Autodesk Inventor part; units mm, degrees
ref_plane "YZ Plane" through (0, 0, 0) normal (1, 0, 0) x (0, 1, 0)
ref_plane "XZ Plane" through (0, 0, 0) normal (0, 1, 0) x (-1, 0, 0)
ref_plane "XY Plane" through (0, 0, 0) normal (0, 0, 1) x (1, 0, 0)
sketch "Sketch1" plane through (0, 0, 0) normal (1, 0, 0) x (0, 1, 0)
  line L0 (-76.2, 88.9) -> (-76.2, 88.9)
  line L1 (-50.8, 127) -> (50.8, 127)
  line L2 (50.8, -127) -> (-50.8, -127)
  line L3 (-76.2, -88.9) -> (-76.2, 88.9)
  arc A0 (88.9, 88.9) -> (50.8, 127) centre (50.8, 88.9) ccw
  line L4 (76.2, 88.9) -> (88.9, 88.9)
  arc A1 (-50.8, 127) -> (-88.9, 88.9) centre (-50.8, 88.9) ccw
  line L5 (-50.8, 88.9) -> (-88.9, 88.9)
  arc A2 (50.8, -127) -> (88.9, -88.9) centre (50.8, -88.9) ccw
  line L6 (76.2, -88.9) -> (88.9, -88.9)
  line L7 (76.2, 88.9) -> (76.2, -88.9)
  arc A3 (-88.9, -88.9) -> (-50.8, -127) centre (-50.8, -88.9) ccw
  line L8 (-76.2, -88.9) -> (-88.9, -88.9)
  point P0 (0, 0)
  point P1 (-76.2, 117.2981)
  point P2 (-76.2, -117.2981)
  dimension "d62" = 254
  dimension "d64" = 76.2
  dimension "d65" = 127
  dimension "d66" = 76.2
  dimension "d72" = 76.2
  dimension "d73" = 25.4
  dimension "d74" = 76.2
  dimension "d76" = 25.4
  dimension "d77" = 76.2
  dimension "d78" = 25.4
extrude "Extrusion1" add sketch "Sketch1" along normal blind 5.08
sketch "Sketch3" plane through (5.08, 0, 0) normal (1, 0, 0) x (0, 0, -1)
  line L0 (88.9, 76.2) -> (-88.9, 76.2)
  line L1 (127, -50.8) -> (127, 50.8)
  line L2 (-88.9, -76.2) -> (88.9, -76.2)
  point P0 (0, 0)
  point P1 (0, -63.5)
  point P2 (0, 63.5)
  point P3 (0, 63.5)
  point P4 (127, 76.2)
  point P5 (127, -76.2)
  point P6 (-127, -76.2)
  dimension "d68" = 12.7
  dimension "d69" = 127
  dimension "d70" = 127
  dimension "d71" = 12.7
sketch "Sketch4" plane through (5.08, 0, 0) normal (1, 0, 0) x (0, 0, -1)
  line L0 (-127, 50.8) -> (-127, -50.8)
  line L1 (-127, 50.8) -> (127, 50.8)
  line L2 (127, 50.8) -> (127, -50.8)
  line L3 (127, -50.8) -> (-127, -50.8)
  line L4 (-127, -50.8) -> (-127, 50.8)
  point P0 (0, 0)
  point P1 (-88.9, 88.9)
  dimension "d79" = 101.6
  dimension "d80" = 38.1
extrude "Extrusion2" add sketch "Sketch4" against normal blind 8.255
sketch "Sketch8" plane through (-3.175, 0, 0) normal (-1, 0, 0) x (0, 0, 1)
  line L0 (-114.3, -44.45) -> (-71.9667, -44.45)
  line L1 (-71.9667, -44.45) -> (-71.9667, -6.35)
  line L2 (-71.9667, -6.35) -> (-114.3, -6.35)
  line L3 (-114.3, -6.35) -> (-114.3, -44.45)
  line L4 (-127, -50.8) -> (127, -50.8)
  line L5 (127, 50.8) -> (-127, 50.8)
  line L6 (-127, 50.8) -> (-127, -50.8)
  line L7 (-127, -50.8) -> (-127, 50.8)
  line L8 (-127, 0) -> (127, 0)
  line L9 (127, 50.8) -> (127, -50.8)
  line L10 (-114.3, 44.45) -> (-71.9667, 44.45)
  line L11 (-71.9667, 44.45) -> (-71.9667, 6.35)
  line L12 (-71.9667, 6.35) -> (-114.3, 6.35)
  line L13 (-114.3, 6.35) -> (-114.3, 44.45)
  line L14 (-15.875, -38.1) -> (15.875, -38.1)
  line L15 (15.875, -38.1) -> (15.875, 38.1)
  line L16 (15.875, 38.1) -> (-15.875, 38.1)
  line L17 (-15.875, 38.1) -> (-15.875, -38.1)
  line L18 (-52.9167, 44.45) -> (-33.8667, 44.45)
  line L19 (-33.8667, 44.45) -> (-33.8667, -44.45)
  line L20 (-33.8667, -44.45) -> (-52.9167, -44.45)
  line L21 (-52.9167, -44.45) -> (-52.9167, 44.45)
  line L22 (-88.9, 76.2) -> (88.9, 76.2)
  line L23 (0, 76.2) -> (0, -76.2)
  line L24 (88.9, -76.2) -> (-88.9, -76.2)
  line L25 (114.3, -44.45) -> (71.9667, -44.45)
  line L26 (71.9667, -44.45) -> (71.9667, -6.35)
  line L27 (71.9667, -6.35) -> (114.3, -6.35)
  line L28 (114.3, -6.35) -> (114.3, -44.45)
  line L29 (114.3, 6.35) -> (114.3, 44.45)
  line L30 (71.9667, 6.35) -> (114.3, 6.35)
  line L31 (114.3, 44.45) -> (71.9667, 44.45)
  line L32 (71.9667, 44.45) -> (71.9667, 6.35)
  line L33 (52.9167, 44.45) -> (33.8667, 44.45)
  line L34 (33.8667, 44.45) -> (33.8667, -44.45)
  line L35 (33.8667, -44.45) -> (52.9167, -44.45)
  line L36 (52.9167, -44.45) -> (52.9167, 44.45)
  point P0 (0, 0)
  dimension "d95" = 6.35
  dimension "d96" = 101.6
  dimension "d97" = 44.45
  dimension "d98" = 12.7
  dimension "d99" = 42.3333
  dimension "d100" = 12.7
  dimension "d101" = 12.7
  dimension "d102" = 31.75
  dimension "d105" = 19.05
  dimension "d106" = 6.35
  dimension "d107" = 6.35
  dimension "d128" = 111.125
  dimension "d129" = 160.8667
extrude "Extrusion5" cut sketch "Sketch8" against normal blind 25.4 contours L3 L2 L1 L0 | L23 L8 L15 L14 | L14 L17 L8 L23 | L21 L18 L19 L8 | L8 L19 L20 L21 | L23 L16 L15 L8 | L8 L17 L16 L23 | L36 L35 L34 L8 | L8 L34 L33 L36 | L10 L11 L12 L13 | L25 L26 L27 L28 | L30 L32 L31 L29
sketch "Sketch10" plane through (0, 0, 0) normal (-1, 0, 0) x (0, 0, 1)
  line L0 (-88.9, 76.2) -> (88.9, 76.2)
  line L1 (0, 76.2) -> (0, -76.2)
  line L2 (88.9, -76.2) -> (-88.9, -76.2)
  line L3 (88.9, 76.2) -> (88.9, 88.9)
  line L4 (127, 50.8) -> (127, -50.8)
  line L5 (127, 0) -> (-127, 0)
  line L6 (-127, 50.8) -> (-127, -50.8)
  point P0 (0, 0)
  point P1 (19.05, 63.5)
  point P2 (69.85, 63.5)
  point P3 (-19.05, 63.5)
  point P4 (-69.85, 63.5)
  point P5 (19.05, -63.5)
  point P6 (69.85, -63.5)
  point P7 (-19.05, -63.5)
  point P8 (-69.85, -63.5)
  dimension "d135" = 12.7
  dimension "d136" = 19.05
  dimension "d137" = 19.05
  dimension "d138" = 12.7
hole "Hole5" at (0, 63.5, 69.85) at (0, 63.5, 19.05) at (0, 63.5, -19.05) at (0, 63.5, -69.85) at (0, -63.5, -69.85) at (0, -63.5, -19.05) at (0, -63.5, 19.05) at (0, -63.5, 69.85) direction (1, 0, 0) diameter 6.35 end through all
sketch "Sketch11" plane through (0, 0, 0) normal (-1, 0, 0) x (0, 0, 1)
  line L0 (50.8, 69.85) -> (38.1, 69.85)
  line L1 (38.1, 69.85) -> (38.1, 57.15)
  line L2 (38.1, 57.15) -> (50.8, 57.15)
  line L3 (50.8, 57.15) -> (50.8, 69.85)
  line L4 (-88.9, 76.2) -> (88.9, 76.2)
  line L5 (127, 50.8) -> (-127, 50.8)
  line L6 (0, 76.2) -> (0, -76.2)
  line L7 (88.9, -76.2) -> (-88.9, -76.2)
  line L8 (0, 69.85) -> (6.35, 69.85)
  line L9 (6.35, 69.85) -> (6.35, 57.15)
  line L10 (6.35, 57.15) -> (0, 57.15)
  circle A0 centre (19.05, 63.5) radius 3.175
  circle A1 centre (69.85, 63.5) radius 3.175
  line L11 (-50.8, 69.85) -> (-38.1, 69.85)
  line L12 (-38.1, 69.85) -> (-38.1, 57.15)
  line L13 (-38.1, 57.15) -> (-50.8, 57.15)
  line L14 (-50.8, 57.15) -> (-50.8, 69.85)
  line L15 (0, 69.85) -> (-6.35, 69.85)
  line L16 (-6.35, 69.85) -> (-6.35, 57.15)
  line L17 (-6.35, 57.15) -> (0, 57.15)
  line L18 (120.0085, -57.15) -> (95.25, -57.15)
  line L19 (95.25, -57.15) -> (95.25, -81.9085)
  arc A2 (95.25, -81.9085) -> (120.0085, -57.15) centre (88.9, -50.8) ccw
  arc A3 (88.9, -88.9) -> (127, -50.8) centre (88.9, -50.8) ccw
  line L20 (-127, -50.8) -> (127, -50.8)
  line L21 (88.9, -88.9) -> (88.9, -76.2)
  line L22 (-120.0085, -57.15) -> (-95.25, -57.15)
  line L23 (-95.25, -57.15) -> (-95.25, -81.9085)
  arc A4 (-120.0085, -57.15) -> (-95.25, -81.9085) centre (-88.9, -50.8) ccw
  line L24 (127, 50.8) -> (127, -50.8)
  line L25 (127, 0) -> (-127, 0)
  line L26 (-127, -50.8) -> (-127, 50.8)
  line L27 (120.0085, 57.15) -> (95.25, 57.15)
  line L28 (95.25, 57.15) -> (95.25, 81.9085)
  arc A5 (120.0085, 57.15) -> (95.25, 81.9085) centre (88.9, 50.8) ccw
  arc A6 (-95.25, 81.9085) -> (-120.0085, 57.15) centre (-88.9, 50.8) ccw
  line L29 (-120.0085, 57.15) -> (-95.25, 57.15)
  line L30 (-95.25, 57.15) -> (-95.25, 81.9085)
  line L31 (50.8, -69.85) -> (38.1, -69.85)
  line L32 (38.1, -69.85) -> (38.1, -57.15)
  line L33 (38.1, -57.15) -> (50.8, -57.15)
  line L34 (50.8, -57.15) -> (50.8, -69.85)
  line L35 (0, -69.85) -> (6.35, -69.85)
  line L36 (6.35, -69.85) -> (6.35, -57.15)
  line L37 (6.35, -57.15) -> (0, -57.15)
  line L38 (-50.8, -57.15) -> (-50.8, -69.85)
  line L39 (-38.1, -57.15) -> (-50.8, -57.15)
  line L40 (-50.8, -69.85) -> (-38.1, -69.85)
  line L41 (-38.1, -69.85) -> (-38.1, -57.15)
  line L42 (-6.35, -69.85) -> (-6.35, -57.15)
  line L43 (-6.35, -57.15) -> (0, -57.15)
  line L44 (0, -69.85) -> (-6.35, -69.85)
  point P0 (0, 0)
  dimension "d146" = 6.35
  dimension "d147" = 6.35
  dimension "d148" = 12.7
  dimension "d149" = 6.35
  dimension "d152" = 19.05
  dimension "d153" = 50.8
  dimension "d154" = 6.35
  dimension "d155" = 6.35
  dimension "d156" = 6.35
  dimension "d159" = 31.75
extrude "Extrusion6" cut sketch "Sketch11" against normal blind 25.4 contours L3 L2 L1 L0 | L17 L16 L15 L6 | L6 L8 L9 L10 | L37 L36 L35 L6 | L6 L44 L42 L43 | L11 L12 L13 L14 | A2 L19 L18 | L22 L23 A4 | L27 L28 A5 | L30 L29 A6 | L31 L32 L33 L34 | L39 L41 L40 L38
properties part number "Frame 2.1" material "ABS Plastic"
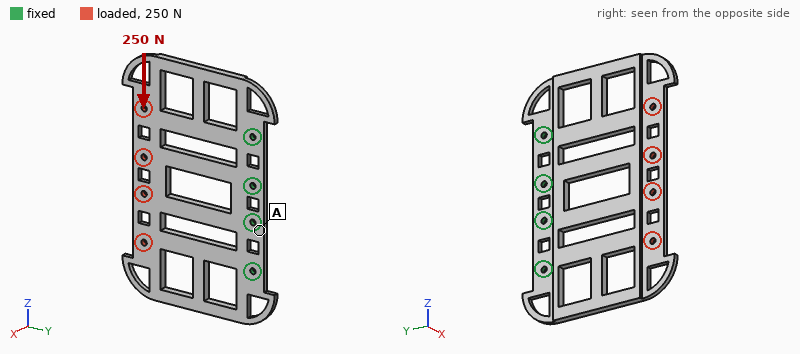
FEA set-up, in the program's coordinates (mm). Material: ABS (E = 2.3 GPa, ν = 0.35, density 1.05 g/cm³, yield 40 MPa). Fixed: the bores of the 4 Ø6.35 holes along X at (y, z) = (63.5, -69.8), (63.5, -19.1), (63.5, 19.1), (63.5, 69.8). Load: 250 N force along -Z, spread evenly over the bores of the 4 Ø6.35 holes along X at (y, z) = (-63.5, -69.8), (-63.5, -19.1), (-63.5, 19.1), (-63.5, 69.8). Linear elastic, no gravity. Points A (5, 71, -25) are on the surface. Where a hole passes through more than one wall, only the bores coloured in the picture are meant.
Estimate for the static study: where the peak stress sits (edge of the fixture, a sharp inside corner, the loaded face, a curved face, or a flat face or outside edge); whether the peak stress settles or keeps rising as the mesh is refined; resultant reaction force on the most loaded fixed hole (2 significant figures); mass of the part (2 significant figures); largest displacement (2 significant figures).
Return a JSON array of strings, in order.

["edge of the fixture", "keeps rising", "210 N", "170 g", "0.83 mm"]
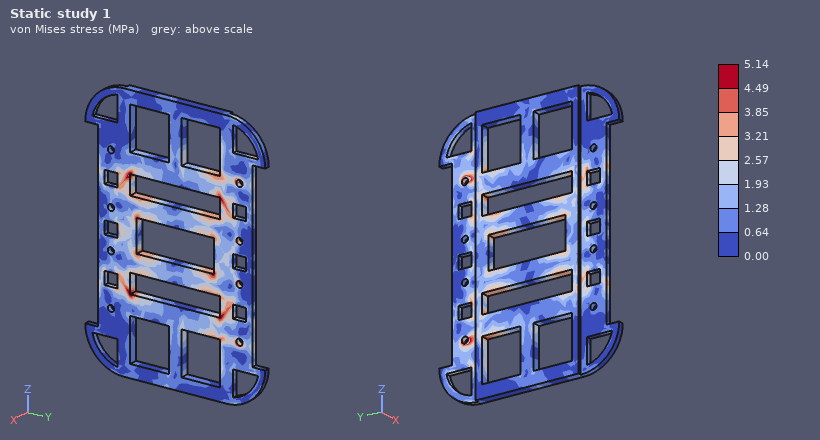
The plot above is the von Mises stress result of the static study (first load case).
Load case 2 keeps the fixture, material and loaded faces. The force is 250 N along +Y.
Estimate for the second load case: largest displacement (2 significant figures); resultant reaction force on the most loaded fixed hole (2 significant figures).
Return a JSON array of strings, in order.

["0.32 mm", "65 N"]
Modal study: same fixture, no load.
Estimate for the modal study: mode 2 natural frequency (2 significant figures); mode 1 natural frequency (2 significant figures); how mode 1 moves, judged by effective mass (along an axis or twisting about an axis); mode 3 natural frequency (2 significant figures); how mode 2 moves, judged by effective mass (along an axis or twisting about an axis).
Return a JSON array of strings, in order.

["100 Hz", "66 Hz", "along X", "200 Hz", "twisting about Y"]
